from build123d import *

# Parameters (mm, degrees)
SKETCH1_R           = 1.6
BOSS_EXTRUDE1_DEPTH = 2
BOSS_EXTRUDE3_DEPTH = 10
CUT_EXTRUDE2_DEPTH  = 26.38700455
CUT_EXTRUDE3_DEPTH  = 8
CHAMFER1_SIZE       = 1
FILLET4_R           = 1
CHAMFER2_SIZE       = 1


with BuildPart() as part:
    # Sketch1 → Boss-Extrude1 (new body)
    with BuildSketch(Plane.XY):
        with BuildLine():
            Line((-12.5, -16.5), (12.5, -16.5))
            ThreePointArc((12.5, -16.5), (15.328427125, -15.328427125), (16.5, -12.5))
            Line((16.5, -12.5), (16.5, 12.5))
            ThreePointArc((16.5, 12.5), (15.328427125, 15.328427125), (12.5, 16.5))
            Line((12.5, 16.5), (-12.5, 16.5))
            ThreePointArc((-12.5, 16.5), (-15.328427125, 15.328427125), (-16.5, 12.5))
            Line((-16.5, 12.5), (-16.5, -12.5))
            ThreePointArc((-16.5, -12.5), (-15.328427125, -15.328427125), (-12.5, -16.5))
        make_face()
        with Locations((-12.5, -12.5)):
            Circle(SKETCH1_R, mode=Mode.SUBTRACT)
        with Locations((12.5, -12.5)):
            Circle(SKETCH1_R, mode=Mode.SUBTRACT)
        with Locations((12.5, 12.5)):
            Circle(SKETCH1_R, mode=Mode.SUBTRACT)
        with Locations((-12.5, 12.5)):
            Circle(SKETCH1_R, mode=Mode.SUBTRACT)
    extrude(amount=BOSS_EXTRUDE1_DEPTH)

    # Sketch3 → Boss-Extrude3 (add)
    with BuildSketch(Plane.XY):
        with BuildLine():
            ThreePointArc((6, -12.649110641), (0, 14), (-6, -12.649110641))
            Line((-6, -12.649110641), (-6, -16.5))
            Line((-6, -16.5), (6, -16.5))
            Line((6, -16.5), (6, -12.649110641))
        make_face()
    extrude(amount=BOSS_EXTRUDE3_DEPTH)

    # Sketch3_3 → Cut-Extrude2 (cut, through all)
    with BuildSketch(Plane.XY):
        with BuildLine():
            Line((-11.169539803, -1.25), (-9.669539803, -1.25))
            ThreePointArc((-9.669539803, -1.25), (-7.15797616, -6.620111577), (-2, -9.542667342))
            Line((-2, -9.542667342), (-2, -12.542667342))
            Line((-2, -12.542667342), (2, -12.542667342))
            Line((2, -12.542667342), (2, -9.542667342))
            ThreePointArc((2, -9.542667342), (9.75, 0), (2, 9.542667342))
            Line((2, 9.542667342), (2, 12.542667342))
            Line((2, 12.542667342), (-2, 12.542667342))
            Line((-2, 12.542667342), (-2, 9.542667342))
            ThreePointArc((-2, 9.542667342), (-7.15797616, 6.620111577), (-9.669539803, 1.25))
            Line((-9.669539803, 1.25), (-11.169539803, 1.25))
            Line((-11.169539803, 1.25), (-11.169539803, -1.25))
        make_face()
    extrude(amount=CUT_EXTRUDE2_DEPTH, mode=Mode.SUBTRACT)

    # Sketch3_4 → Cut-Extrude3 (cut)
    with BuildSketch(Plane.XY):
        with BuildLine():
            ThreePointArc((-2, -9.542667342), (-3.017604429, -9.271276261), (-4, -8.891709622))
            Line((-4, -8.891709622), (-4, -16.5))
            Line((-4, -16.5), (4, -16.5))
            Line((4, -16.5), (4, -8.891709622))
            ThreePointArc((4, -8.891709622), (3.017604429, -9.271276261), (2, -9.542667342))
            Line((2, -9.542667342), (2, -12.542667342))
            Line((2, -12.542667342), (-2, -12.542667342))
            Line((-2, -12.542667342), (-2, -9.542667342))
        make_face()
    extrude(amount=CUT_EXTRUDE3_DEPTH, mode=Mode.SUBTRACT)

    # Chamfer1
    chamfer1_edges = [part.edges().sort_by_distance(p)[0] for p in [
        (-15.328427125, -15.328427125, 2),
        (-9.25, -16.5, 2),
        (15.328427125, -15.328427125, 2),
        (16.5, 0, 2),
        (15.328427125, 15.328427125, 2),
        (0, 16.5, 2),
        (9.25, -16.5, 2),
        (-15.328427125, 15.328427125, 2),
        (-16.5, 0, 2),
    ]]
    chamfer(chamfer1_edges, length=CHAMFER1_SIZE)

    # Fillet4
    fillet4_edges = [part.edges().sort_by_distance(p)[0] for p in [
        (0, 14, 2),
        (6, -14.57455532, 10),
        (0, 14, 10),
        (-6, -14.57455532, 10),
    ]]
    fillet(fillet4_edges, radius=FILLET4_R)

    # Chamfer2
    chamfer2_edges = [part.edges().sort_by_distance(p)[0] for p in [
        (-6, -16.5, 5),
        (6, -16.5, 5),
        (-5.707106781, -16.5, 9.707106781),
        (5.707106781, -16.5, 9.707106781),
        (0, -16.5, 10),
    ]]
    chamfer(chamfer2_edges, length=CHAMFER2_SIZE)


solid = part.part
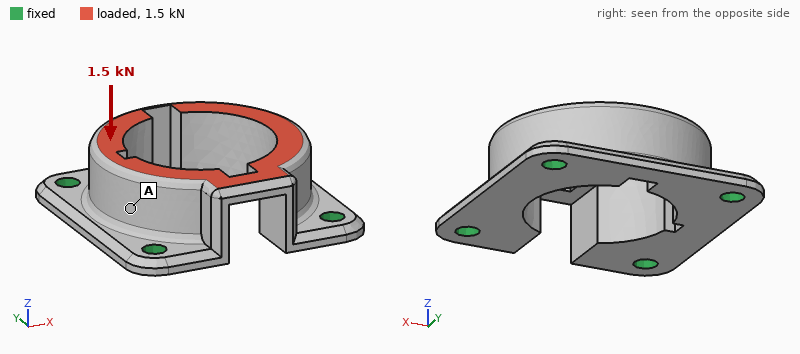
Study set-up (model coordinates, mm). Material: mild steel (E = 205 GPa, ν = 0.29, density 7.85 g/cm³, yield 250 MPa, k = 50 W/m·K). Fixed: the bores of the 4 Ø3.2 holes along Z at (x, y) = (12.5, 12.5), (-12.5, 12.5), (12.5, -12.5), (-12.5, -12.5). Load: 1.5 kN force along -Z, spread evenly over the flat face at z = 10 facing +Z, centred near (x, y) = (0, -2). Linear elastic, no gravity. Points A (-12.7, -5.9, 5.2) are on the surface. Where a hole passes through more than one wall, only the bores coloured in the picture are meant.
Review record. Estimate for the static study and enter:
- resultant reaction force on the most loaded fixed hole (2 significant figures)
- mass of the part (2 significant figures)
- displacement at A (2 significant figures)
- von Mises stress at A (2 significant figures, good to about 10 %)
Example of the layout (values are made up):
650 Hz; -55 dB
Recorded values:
490 N; 28 g; 2.7 µm; 15 MPa
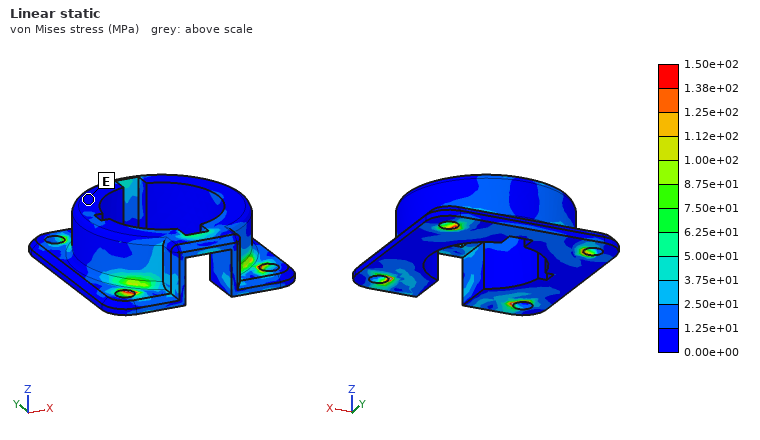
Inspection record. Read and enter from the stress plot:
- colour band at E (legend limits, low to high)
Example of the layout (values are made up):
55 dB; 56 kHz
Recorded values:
0.00e+00 to 1.25e+01 MPa
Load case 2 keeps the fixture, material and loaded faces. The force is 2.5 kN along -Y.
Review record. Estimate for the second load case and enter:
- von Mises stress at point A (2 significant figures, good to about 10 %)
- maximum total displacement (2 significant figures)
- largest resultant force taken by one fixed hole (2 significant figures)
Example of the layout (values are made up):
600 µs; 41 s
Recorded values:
19 MPa; 12 µm; 820 N
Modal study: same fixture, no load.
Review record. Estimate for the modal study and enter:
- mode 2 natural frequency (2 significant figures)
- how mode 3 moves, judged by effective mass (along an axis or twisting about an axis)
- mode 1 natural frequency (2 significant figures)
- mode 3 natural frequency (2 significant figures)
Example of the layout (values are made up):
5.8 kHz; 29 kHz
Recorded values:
18 kHz; along Z; 18 kHz; 22 kHz
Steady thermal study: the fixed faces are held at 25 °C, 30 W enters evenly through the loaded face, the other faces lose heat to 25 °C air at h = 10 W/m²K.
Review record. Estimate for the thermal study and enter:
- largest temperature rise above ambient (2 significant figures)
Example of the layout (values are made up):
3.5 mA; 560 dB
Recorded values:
65 K
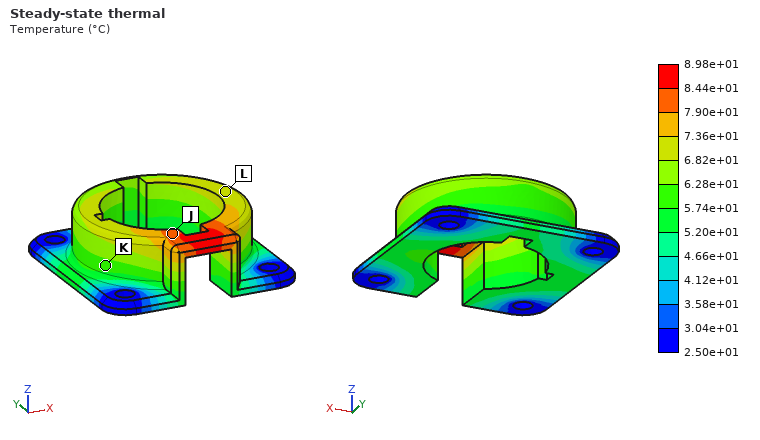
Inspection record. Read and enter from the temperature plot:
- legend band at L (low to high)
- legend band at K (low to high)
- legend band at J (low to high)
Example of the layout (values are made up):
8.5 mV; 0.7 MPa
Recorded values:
6.82e+01 to 7.36e+01 °C; 5.74e+01 to 6.28e+01 °C; 7.90e+01 to 8.44e+01 °C
